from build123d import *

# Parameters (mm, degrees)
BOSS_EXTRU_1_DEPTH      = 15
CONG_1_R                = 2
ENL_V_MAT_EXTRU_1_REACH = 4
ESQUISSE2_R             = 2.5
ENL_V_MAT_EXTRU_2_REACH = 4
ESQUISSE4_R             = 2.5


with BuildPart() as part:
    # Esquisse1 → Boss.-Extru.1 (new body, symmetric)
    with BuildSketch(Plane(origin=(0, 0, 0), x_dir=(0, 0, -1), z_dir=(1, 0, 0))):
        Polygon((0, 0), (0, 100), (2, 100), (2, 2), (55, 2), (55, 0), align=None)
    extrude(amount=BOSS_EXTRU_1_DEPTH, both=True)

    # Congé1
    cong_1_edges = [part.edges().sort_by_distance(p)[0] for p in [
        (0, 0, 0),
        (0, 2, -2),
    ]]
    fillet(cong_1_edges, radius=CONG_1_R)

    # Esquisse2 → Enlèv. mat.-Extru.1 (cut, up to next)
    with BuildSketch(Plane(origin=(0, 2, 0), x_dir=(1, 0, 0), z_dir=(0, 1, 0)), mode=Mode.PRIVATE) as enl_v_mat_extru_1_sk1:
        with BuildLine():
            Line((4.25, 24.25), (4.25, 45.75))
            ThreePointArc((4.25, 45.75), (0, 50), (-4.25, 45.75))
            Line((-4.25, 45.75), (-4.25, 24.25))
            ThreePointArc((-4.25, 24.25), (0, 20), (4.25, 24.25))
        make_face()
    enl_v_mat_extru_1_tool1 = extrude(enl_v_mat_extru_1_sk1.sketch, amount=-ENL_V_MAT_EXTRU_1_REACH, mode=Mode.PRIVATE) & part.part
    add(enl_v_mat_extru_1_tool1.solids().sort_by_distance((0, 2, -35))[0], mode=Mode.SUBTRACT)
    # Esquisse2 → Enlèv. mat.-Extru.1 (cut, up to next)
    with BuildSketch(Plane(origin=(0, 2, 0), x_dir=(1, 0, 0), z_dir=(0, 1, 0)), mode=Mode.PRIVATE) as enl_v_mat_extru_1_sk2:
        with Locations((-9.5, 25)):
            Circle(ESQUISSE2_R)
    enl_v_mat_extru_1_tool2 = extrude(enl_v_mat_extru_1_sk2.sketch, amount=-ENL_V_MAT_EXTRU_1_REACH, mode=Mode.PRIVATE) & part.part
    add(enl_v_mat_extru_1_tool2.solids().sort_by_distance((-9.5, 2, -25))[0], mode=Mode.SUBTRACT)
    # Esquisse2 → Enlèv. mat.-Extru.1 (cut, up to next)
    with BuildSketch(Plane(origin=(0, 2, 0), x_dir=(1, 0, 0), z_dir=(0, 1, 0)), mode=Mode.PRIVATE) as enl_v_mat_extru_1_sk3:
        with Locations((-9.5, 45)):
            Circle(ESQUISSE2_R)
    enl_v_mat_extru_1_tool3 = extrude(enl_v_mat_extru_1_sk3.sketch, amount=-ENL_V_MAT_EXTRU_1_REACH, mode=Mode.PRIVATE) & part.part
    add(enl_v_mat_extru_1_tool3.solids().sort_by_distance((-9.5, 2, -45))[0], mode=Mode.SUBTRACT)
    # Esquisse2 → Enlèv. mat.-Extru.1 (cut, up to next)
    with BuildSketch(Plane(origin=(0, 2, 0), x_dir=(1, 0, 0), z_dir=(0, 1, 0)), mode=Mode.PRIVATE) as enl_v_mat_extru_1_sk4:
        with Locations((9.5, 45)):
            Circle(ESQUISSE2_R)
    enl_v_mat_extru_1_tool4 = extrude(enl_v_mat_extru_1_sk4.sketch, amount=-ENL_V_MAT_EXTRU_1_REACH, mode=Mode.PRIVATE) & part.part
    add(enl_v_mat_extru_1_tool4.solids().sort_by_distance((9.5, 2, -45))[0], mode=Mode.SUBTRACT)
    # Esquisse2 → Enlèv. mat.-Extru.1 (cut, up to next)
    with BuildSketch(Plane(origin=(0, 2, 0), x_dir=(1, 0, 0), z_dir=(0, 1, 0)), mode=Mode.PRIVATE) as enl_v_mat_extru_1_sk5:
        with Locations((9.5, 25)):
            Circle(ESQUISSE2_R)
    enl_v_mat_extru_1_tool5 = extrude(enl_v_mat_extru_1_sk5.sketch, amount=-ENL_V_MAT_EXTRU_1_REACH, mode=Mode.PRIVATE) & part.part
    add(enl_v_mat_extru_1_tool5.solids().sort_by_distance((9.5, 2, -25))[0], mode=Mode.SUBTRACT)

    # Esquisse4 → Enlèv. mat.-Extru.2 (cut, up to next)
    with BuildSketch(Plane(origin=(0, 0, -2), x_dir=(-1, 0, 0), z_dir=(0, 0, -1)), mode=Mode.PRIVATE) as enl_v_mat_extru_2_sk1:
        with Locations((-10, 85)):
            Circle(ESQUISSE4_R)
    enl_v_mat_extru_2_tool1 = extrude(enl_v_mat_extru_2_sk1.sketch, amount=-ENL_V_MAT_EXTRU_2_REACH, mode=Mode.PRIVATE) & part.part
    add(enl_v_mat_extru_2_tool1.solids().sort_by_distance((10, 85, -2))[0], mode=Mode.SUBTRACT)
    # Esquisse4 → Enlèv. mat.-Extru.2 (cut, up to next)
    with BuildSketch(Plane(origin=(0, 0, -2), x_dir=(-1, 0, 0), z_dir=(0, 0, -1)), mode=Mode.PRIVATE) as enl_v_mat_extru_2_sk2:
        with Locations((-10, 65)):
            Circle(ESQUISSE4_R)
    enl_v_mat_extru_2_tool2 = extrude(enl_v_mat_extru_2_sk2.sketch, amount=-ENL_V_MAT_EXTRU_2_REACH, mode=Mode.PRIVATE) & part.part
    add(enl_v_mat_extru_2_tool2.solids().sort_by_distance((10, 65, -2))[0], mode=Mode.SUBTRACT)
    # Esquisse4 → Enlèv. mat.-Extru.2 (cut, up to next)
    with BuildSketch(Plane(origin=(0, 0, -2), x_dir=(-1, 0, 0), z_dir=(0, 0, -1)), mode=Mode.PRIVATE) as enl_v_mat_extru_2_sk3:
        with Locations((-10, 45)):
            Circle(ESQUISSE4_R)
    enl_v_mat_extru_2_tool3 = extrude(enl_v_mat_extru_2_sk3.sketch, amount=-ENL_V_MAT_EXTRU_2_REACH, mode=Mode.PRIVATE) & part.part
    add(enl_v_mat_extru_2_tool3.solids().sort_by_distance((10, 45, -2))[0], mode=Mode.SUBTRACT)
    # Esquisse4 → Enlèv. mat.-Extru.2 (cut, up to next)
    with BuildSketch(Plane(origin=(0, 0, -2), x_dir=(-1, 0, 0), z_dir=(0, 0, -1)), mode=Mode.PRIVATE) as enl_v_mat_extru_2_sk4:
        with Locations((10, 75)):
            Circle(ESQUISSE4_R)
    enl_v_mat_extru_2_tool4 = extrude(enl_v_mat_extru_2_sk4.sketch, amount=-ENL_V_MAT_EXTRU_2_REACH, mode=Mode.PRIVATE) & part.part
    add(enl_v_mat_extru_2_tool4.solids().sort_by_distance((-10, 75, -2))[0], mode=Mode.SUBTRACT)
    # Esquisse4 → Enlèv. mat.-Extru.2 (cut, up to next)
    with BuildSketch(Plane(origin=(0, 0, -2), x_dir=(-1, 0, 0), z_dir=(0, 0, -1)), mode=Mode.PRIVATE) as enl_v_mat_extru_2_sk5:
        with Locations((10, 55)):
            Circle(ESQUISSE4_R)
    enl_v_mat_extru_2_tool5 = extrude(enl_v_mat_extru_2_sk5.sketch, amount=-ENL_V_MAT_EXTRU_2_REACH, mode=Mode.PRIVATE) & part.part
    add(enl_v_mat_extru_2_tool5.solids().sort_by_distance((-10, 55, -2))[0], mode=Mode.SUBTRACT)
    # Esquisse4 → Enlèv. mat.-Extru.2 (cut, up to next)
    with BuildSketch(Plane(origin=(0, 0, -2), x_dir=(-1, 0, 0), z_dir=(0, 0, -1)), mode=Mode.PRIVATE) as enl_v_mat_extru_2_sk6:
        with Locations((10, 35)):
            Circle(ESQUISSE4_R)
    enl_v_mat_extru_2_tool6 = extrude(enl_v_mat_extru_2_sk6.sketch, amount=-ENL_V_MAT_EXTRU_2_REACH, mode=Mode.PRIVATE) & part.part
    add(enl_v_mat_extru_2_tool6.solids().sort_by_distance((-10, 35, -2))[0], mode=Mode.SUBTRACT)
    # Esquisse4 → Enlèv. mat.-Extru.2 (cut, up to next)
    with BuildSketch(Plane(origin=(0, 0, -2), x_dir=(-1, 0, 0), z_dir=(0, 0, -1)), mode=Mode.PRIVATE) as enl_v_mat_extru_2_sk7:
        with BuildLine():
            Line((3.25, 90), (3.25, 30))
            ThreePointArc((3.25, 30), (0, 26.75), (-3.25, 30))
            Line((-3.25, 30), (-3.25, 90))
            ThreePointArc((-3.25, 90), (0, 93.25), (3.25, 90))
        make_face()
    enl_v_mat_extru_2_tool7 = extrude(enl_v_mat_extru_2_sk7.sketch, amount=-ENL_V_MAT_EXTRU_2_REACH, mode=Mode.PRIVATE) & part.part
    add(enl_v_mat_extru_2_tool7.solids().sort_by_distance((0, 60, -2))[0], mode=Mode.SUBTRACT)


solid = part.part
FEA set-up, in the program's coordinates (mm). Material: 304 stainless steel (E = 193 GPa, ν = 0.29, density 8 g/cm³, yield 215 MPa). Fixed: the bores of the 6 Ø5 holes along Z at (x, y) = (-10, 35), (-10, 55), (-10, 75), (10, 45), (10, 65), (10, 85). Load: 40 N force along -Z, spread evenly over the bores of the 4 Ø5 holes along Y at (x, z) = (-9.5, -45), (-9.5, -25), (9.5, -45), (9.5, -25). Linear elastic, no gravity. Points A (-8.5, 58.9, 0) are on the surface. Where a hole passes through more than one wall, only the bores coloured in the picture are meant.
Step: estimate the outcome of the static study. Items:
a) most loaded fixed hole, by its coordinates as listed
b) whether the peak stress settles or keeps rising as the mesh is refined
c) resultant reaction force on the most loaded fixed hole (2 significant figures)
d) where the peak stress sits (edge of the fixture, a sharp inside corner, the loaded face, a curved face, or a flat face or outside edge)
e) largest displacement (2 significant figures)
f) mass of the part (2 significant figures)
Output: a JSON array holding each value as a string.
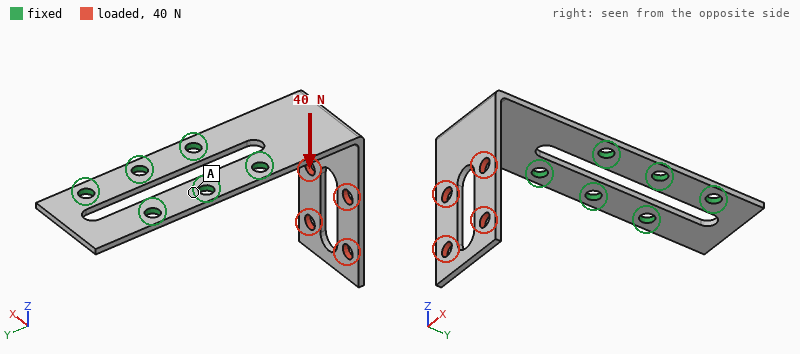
["(-10, 35)", "keeps rising", "44 N", "edge of the fixture", "0.43 mm", "60 g"]
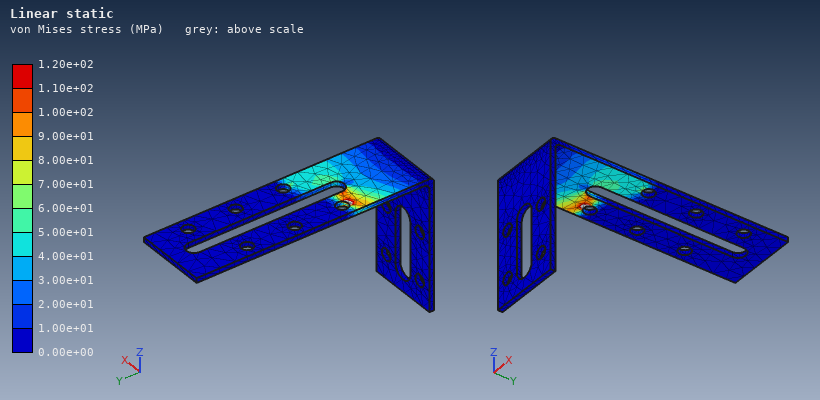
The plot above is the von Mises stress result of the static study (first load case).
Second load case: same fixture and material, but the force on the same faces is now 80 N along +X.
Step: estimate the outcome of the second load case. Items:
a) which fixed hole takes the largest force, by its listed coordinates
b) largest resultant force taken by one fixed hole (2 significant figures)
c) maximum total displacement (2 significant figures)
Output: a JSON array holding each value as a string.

["(-10, 35)", "150 N", "0.79 mm"]
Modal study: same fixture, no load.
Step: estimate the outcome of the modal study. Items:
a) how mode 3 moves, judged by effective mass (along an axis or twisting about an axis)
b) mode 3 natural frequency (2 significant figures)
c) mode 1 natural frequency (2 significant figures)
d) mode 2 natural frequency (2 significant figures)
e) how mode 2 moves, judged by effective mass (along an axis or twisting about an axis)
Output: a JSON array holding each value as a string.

["along Z", "830 Hz", "290 Hz", "500 Hz", "along X"]
